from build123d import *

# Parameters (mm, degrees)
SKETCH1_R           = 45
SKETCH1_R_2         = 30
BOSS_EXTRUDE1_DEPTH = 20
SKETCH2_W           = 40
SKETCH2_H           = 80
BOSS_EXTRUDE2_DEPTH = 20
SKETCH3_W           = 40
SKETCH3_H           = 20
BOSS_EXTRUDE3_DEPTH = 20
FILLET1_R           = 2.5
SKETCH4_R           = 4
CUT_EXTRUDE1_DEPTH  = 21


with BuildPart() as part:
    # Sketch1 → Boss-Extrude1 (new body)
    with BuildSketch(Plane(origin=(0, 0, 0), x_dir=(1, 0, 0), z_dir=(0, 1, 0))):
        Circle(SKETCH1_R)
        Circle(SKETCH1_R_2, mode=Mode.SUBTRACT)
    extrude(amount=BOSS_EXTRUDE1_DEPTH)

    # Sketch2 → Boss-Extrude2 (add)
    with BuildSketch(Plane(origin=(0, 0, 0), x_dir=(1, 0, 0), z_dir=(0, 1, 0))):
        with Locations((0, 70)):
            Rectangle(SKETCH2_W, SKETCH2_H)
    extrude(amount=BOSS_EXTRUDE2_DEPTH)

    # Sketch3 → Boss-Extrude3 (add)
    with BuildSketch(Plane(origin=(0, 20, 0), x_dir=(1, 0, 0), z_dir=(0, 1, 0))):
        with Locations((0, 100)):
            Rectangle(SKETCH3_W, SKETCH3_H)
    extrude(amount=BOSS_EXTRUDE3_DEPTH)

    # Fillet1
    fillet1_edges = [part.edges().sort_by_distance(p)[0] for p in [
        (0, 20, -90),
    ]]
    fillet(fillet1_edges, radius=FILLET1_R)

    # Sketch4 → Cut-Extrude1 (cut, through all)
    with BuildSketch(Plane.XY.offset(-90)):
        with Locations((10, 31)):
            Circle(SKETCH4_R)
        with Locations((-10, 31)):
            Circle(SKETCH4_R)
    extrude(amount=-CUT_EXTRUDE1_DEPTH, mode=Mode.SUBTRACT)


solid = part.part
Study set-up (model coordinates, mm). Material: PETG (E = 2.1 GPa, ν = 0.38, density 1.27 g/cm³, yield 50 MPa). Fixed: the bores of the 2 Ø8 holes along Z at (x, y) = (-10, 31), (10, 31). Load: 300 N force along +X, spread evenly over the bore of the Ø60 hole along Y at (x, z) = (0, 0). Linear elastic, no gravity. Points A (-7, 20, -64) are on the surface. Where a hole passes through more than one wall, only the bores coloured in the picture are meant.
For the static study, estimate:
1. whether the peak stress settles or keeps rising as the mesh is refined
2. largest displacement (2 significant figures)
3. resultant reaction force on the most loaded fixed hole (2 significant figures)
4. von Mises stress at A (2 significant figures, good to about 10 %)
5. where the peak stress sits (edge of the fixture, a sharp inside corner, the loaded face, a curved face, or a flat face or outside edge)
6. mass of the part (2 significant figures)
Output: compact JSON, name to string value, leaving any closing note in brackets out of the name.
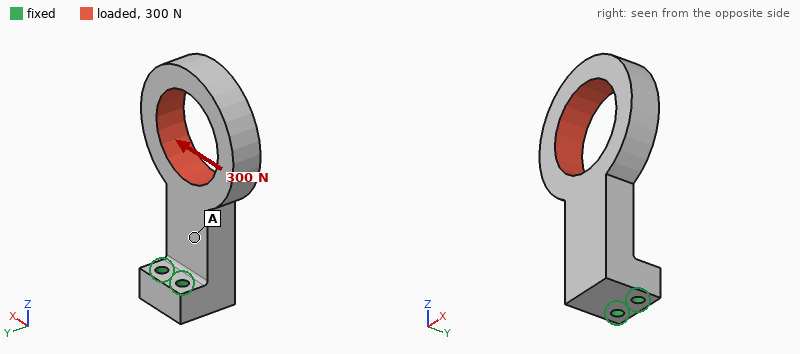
{"whether the peak stress settles or keeps rising as the mesh is refined": "keeps rising", "largest displacement": "1.9 mm", "resultant reaction force on the most loaded fixed hole": "900 N", "von Mises stress at A": "1.8 MPa", "where the peak stress sits": "edge of the fixture", "mass of the part": "180 g"}
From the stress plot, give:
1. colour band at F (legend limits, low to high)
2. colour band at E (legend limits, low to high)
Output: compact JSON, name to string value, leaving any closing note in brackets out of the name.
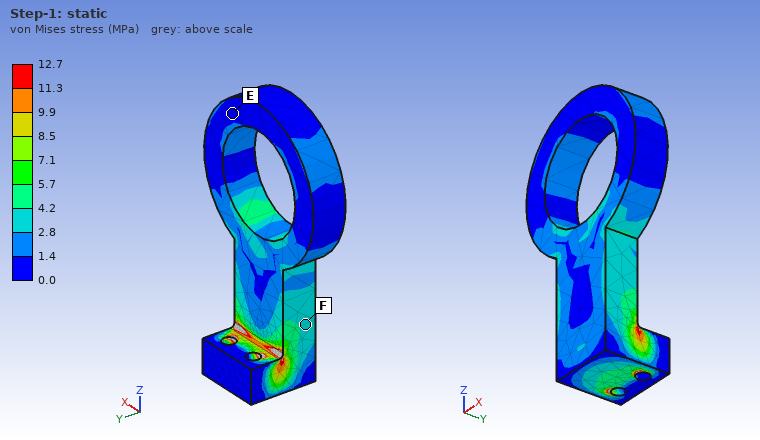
{"colour band at F": "2.8 to 4.2 MPa", "colour band at E": "0.0 to 1.4 MPa"}
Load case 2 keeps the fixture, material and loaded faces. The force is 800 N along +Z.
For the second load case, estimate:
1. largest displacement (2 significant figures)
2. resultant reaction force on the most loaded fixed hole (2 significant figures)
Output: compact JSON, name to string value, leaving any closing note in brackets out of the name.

{"largest displacement": "0.57 mm", "resultant reaction force on the most loaded fixed hole": "400 N"}
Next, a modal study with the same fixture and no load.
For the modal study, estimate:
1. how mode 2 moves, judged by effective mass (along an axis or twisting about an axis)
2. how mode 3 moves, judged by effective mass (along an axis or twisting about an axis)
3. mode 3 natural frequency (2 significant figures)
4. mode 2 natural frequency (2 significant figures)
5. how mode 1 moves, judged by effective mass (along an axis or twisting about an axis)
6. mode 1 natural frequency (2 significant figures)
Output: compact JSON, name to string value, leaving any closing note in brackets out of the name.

{"how mode 2 moves, judged by effective mass": "along X", "how mode 3 moves, judged by effective mass": "twisting about Z", "mode 3 natural frequency": "480 Hz", "mode 2 natural frequency": "240 Hz", "how mode 1 moves, judged by effective mass": "along Y", "mode 1 natural frequency": "160 Hz"}
